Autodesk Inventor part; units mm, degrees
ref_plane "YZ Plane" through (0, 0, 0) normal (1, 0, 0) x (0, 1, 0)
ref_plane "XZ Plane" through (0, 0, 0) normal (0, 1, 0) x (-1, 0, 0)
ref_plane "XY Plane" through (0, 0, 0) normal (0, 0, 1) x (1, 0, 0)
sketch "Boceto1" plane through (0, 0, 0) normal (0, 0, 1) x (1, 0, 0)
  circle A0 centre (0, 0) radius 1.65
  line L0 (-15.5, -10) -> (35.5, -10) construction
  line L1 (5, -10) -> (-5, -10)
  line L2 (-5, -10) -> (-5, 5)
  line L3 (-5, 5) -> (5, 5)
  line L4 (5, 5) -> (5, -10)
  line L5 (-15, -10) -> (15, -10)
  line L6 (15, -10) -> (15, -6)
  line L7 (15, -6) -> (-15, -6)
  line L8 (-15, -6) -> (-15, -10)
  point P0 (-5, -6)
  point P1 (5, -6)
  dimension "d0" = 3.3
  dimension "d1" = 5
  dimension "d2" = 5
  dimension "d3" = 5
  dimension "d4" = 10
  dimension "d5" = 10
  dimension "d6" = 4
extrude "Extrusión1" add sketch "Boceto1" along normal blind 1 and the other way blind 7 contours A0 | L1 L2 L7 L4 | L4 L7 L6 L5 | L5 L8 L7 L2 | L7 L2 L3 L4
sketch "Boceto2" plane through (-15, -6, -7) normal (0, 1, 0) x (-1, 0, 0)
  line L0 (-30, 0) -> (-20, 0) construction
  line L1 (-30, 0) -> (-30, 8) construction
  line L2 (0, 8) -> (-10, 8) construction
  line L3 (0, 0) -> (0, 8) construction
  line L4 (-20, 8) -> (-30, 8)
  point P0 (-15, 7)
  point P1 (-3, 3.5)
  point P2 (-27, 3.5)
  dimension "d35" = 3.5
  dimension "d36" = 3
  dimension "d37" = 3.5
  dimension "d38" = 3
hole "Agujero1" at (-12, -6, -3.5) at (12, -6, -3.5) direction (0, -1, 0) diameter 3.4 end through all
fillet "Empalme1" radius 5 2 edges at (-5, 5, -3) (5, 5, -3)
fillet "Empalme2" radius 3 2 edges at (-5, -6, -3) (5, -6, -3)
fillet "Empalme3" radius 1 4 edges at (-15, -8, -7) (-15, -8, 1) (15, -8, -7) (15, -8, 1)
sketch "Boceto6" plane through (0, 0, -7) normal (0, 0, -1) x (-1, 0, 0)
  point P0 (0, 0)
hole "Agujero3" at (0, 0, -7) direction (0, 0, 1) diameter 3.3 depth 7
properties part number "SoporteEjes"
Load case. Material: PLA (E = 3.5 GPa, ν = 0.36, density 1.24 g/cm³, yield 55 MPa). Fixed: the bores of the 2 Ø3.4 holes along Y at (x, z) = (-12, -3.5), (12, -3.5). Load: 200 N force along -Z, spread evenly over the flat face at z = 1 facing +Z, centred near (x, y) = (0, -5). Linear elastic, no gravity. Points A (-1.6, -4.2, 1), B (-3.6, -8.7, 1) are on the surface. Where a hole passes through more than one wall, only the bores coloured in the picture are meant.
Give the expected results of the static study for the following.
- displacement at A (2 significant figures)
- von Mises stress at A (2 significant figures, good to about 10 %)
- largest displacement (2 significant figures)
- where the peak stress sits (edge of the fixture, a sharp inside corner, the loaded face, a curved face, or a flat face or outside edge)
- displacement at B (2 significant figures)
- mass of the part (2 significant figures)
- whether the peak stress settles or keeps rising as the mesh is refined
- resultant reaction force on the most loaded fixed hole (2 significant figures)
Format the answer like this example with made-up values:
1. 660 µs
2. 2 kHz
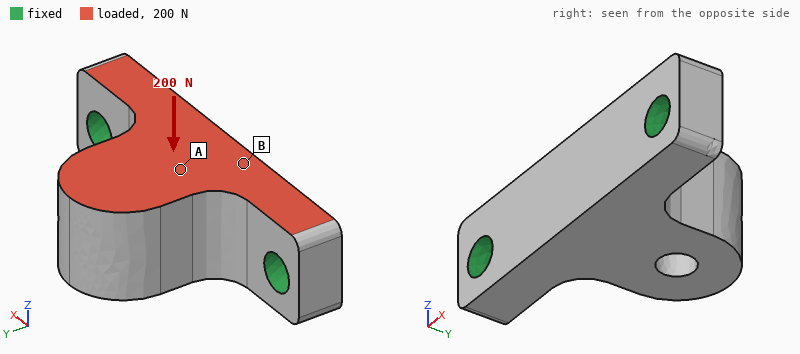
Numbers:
1. 0.091 mm
2. 3.4 MPa
3. 0.20 mm
4. edge of the fixture
5. 0.050 mm
6. 2.0 g
7. keeps rising
8. 100 N
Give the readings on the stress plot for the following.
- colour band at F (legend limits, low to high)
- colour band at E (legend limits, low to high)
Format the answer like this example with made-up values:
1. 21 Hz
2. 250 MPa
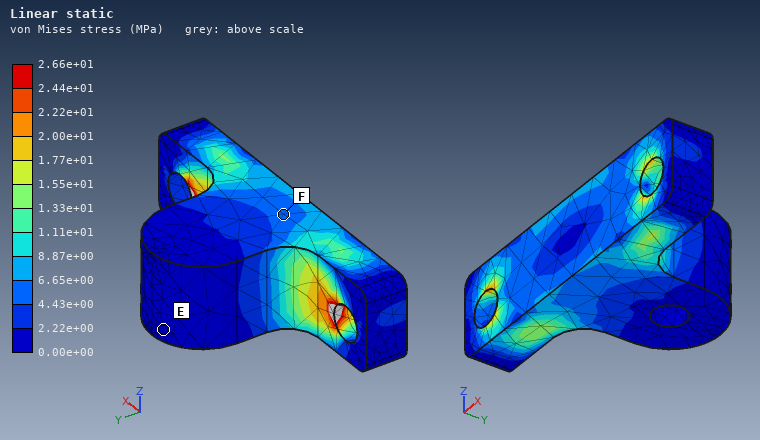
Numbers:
1. 4.43e+00 to 6.65e+00 MPa
2. 0.00e+00 to 2.22e+00 MPa
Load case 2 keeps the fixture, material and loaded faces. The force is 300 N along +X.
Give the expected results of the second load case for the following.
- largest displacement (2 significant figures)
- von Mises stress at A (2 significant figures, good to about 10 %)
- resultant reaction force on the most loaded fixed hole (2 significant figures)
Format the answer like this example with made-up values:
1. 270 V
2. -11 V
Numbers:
1. 58 µm
2. 7.0 MPa
3. 170 N
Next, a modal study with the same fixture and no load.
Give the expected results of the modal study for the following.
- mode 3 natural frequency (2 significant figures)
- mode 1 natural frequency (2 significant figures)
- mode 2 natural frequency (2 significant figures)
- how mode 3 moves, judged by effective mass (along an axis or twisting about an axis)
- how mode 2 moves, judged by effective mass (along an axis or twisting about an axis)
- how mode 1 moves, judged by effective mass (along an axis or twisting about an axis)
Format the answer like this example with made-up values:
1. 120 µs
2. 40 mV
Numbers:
1. 11 kHz
2. 4400 Hz
3. 9600 Hz
4. along X
5. along Y
6. along Z
